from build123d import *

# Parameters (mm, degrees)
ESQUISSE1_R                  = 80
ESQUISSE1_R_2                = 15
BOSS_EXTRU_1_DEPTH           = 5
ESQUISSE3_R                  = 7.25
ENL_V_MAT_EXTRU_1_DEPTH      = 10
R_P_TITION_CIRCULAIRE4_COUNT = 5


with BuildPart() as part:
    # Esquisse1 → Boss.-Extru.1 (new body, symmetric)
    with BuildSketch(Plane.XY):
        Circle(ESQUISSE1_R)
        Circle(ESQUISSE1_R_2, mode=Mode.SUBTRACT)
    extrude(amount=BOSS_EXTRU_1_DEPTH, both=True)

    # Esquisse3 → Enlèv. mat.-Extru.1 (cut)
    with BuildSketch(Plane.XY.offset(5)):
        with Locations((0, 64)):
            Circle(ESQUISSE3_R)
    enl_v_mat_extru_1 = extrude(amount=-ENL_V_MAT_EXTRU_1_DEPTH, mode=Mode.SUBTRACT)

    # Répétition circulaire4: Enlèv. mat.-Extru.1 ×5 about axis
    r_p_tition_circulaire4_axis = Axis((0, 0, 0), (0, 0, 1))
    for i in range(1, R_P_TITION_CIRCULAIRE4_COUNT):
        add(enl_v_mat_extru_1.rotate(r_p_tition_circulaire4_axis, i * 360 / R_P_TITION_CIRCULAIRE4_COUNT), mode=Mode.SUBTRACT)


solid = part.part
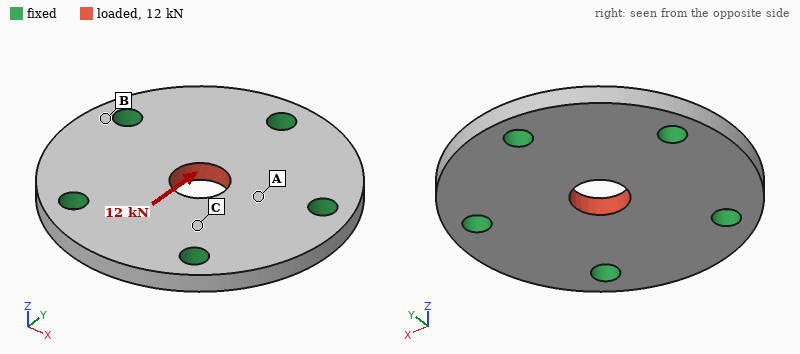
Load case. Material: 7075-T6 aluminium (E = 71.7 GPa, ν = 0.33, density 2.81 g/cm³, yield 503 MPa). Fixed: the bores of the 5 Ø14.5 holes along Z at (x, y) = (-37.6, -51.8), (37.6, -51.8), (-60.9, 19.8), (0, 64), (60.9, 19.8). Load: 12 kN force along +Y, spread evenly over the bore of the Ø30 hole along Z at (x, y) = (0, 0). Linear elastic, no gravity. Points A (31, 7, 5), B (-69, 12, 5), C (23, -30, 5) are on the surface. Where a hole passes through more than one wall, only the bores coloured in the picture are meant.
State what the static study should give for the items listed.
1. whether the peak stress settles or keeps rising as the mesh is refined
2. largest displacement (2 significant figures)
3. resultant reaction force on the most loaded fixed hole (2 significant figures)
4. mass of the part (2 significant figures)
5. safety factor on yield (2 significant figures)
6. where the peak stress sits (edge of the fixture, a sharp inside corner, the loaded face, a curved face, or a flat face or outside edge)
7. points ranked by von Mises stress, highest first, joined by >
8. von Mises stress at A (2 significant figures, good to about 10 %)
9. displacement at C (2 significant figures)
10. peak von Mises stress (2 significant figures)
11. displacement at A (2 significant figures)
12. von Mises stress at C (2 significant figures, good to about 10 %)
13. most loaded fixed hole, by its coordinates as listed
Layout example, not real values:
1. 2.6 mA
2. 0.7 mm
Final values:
1. settles
2. 7.5 µm
3. 3.5 kN
4. 520 g
5. 23
6. the loaded face
7. C > A > B
8. 4.9 MPa
9. 3.1 µm
10. 22 MPa
11. 3.2 µm
12. 9.9 MPa
13. (0, 64)
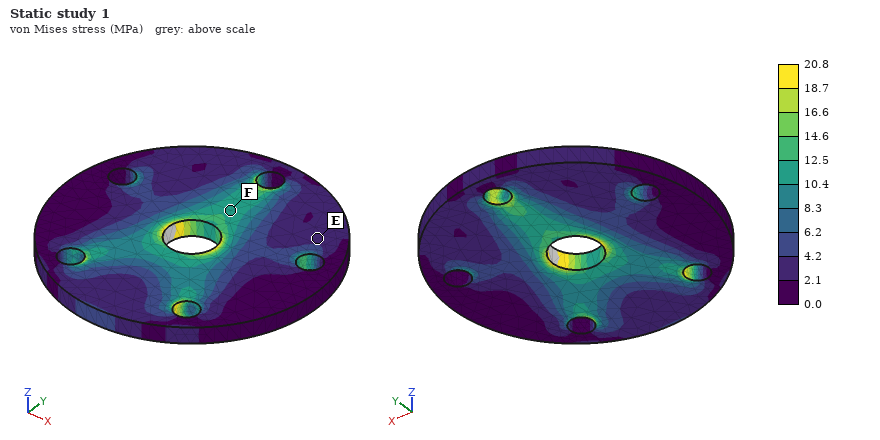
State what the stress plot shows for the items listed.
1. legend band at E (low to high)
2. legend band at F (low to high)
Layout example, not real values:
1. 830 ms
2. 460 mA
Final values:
1. 2.1 to 4.2 MPa
2. 10.4 to 12.5 MPa
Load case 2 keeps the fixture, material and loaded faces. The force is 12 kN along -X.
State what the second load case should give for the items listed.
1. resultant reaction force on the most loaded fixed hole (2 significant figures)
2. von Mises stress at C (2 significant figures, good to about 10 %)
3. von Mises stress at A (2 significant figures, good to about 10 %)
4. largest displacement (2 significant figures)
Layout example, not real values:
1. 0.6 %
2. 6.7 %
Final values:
1. 3.4 kN
2. 7.4 MPa
3. 11 MPa
4. 7.5 µm
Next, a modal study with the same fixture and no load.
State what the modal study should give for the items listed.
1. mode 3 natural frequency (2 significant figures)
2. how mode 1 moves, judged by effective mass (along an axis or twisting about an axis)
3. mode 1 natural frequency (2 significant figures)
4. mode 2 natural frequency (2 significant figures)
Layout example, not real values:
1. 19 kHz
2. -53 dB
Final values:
1. 8100 Hz
2. along Z
3. 5700 Hz
4. 8100 Hz
